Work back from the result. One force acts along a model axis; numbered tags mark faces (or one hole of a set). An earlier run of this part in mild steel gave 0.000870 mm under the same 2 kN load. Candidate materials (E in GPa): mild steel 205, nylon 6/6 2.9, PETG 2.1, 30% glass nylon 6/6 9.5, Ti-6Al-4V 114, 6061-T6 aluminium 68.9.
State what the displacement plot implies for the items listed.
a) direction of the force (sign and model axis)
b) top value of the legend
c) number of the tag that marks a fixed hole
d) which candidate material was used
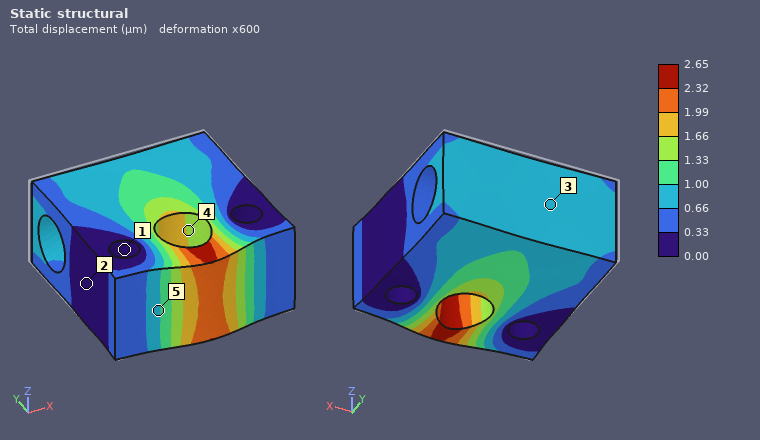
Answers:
-Y
2.65 µm
1
6061-T6 aluminium
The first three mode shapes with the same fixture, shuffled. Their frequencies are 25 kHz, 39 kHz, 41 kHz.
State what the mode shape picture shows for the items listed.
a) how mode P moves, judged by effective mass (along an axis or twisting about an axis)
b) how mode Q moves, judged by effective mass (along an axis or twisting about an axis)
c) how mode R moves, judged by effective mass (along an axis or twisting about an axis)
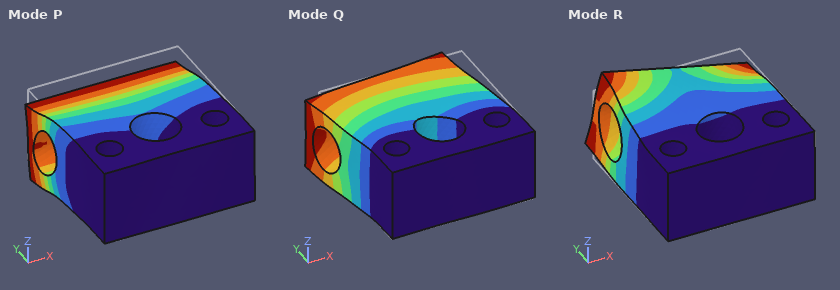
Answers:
along Z
along X
twisting about Y
